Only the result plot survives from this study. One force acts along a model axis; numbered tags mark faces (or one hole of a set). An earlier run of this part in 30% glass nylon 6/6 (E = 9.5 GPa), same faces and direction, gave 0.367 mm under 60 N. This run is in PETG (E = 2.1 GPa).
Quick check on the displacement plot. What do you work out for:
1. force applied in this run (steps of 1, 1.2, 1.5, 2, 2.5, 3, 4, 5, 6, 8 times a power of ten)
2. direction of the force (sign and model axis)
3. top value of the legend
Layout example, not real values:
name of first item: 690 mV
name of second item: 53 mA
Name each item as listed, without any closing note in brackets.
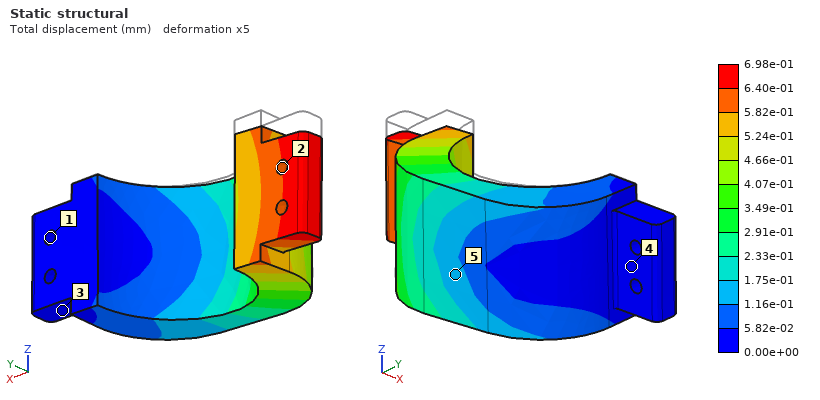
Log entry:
force applied in this run: 25 N
direction of the force: -Z
top value of the legend: 6.98e-01 mm
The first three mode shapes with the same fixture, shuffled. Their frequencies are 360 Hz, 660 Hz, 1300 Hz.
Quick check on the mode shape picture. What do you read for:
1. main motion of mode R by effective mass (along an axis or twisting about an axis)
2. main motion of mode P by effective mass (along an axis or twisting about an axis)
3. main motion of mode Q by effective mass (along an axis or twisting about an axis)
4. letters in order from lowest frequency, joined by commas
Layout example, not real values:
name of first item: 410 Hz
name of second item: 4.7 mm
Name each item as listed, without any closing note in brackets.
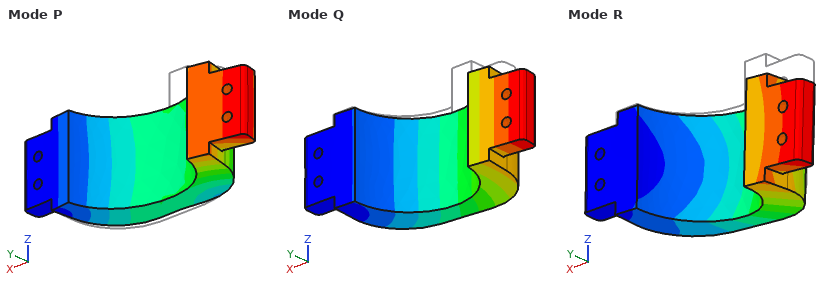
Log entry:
main motion of mode R by effective mass: along Z
main motion of mode P by effective mass: along X
main motion of mode Q by effective mass: along Y
letters in order from lowest frequency, joined by commas: Q, R, P
